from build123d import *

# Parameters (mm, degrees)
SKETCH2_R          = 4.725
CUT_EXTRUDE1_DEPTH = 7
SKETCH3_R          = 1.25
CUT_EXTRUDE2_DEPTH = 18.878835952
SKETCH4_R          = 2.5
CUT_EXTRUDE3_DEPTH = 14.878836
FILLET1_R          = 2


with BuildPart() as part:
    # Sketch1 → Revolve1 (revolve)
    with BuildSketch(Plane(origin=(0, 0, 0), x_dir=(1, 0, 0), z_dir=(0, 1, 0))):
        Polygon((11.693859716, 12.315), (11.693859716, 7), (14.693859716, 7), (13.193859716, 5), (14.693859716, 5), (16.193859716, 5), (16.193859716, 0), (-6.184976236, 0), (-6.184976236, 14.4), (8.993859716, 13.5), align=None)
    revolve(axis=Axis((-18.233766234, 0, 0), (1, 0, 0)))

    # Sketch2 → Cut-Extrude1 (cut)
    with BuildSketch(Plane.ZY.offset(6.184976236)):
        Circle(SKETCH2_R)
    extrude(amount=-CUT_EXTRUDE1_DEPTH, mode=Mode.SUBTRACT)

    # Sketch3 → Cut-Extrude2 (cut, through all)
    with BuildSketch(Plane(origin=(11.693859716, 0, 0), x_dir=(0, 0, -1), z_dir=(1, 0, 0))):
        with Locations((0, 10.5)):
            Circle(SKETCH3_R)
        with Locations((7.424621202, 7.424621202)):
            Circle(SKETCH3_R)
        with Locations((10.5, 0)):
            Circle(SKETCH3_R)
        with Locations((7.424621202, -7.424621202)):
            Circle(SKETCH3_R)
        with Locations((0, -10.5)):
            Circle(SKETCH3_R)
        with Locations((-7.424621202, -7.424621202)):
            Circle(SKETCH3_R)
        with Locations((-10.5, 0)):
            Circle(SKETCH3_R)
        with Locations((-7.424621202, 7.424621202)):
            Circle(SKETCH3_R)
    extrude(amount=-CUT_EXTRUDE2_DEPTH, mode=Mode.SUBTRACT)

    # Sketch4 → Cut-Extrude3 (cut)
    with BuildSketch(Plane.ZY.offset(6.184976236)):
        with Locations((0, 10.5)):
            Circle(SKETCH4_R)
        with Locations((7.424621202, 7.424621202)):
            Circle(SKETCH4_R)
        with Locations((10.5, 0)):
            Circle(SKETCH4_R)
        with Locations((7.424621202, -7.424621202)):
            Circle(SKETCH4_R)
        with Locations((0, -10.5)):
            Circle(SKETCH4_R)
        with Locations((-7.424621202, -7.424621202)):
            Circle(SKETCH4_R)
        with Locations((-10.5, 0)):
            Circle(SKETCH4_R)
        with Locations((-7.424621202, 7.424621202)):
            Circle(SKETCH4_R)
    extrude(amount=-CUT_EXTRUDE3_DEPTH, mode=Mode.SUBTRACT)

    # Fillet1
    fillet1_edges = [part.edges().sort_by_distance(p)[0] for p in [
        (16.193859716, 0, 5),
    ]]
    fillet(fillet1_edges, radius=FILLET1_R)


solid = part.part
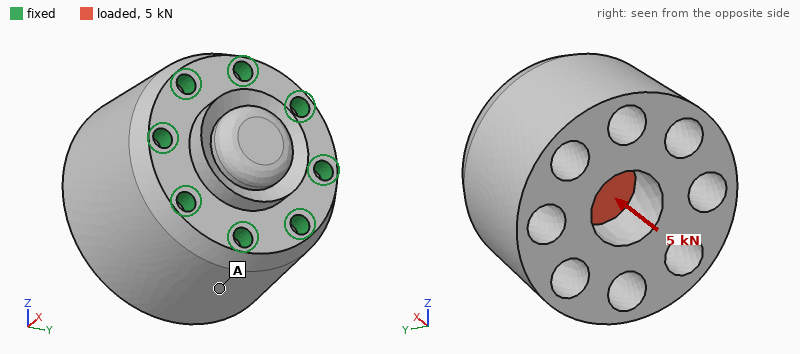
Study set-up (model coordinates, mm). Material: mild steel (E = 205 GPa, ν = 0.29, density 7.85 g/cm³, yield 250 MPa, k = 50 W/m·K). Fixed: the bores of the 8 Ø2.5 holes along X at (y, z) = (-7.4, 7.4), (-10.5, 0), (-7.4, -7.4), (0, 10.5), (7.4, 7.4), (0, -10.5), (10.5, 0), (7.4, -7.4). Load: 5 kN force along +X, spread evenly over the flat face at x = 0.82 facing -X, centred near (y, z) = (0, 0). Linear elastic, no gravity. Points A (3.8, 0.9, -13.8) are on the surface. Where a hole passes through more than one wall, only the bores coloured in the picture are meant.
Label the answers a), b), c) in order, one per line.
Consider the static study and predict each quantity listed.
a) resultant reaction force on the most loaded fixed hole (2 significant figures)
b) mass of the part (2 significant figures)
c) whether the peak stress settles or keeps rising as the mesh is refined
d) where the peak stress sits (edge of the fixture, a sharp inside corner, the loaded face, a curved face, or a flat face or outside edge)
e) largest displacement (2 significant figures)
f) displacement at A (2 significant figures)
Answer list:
a) 660 N
b) 65 g
c) keeps rising
d) edge of the fixture
e) 3.0 µm
f) 0.57 µm
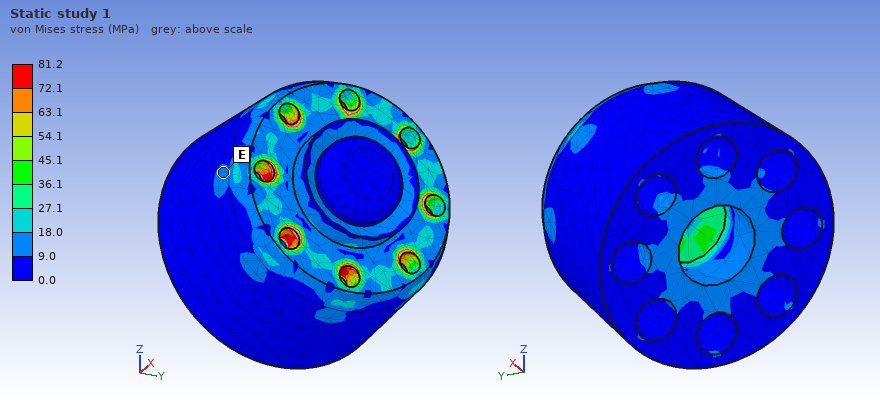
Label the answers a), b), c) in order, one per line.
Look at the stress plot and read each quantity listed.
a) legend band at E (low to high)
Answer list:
a) 9.0 to 18.0 MPa
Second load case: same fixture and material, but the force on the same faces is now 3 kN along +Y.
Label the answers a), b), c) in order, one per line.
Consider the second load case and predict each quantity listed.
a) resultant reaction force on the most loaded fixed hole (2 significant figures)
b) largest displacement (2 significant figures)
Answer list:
a) 810 N
b) 3.0 µm
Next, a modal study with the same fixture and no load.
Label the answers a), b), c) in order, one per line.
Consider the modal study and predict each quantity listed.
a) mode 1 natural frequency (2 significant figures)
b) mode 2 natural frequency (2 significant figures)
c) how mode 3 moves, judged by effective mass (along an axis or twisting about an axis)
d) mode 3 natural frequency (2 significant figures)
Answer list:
a) 27 kHz
b) 27 kHz
c) twisting about X
d) 38 kHz
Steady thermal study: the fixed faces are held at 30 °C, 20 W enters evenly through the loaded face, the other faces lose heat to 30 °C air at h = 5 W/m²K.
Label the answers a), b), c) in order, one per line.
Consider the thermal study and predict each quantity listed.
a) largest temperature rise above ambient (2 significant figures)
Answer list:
a) 27 K
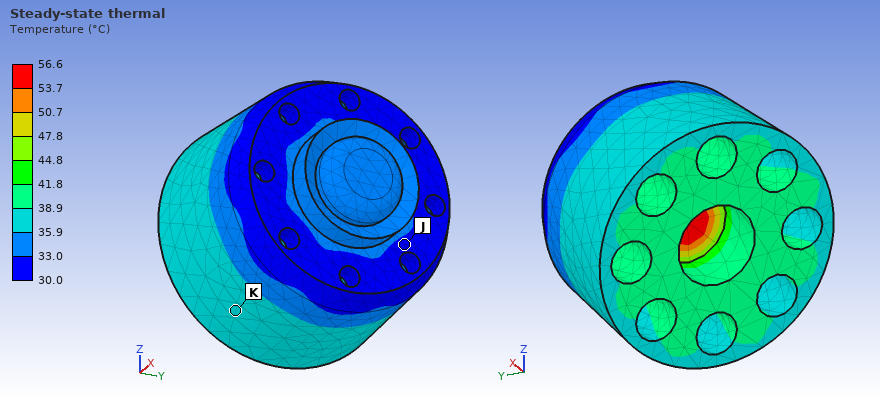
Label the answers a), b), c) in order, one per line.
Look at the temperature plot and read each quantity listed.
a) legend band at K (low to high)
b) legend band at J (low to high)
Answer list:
a) 35.9 to 38.9 °C
b) 30.0 to 33.0 °C
